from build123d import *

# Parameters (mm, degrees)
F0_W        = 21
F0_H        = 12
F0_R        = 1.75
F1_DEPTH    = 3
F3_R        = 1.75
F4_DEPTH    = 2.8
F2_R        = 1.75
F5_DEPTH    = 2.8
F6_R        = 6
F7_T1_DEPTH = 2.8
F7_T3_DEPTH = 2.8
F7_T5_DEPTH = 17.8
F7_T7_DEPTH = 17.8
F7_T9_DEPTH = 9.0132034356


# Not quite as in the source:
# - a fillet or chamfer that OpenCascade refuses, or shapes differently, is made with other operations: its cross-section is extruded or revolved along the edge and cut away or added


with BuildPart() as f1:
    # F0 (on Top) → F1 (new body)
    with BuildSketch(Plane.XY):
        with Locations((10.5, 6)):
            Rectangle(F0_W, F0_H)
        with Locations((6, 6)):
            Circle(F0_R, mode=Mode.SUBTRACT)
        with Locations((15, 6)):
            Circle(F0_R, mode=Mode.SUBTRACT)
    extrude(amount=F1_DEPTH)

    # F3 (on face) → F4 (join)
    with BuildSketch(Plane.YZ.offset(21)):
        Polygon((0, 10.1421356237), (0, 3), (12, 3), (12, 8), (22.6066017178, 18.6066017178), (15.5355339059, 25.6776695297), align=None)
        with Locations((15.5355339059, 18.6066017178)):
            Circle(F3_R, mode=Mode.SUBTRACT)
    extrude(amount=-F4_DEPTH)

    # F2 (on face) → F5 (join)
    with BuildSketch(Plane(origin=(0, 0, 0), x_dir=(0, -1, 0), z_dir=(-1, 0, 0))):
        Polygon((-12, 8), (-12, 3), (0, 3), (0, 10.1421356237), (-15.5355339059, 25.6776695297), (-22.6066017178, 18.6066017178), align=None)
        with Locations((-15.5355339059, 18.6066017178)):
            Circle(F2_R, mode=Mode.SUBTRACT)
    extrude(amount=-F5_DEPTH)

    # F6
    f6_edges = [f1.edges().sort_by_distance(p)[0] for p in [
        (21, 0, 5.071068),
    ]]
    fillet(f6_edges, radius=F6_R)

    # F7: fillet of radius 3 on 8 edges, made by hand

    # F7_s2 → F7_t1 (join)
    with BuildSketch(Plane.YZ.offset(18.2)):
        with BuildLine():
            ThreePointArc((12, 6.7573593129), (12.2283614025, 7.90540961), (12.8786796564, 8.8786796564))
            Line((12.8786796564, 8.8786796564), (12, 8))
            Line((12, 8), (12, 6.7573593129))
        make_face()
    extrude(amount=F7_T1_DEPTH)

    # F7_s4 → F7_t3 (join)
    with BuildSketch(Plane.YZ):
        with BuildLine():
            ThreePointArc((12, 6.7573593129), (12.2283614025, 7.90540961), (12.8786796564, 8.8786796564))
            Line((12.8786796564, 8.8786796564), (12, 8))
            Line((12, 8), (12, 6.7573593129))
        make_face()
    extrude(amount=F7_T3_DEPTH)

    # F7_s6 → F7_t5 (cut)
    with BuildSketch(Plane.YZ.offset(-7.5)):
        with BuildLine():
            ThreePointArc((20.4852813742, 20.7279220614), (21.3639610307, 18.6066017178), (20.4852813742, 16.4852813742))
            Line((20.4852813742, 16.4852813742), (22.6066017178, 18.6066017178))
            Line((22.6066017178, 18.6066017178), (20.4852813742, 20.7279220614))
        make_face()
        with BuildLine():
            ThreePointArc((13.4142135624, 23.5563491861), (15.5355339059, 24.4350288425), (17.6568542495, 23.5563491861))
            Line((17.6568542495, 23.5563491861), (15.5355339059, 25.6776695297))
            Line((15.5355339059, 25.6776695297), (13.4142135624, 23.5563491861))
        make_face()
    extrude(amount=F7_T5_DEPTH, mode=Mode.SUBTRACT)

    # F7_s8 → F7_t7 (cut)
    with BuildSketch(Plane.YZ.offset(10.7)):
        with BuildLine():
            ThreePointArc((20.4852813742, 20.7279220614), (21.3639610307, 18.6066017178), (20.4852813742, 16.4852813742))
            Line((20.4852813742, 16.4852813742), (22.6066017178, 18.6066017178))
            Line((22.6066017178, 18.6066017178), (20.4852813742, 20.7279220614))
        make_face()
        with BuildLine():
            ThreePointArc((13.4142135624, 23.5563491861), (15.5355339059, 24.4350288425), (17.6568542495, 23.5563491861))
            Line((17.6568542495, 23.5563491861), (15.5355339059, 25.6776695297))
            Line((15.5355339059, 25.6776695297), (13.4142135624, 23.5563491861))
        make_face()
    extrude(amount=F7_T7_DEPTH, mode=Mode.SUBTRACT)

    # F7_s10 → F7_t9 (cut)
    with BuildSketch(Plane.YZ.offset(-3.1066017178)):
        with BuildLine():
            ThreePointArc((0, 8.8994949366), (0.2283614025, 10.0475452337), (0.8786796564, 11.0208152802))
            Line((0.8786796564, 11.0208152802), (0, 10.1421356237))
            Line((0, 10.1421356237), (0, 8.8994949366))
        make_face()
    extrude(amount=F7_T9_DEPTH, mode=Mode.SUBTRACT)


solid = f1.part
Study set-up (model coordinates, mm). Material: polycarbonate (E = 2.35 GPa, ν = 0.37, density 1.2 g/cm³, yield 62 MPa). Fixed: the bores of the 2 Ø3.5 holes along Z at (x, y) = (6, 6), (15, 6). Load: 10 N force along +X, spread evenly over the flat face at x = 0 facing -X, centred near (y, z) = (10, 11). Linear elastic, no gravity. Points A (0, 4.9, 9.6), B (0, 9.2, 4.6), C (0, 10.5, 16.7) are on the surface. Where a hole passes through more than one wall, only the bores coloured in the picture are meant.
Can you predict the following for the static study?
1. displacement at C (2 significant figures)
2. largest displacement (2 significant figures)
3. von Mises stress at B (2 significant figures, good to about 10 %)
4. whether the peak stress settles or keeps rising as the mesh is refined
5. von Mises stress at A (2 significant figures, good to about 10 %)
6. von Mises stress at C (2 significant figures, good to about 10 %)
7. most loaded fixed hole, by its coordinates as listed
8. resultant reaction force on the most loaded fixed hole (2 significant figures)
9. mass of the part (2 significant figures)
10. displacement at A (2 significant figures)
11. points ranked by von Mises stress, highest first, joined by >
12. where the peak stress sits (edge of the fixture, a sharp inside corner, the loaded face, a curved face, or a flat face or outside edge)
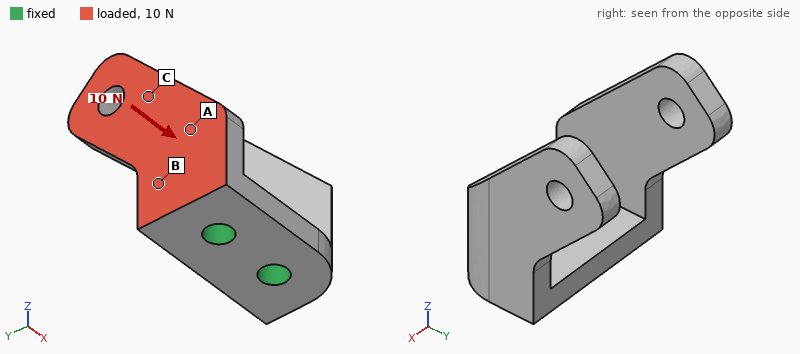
0.22 mm
0.40 mm
4.9 MPa
keeps rising
2.8 MPa
1.1 MPa
(6, 6)
9.7 N
2.4 g
0.082 mm
B > A > C
edge of the fixture
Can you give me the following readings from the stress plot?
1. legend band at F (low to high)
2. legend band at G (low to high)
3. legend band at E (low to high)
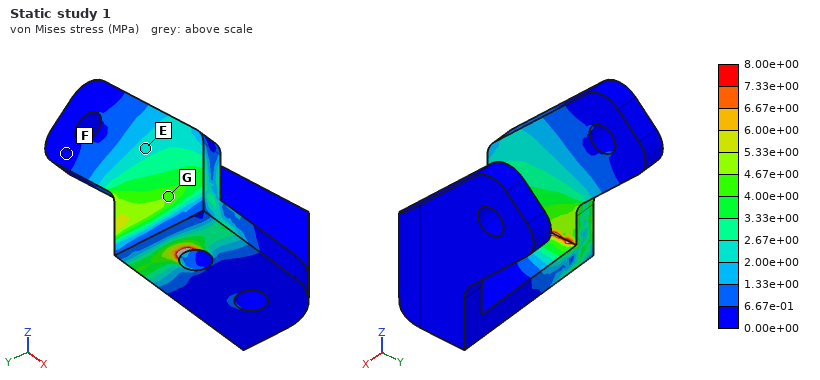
0.00e+00 to 6.67e-01 MPa
4.00e+00 to 4.67e+00 MPa
2.00e+00 to 2.67e+00 MPa
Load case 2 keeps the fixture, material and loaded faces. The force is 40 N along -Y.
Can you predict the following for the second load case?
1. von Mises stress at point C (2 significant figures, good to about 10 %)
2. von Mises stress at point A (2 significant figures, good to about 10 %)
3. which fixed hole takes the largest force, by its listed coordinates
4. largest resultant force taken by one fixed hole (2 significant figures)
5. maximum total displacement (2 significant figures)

2.1 MPa
3.0 MPa
(6, 6)
52 N
0.38 mm
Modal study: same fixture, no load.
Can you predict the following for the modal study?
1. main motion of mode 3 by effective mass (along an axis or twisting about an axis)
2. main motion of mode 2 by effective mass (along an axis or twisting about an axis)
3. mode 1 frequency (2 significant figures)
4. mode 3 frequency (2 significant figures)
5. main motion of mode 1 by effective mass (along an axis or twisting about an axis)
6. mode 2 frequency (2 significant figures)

along Y
along X
980 Hz
1900 Hz
along X
1100 Hz
